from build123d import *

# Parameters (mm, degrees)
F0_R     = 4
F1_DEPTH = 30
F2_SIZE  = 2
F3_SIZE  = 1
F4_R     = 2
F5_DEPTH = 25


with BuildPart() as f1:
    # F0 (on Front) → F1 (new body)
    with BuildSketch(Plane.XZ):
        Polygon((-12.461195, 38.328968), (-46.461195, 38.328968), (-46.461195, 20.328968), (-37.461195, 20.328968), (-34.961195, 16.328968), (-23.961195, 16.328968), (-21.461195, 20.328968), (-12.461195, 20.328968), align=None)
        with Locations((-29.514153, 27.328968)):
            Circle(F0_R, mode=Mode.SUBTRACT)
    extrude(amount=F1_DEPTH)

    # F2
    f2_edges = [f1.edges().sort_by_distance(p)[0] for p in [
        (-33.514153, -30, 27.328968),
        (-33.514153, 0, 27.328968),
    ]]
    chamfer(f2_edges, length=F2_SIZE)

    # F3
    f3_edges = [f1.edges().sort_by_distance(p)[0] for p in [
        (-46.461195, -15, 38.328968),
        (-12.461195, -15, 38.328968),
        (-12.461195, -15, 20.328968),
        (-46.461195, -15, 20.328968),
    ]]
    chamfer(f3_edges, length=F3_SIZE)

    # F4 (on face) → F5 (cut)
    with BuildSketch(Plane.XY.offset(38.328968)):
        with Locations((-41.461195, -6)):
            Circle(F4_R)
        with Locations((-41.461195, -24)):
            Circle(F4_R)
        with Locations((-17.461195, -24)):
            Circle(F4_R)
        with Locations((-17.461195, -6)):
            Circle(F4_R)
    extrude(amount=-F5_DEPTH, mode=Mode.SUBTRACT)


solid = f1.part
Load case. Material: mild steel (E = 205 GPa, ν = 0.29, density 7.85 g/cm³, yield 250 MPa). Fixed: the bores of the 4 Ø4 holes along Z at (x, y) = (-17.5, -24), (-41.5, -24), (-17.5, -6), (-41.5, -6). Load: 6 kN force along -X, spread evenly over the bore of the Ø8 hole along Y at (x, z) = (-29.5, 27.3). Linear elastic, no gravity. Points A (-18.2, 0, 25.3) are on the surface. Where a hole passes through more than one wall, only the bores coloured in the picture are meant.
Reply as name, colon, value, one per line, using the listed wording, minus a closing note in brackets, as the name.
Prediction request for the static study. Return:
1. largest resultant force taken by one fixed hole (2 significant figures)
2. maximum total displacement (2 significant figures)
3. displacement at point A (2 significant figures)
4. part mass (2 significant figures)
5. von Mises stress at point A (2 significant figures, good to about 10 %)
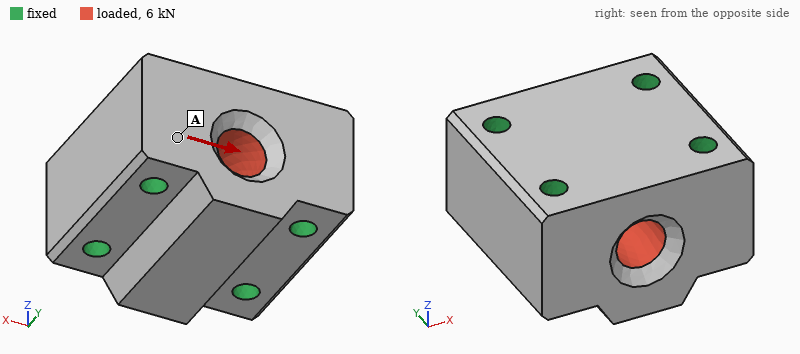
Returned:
largest resultant force taken by one fixed hole: 1.5 kN
maximum total displacement: 0.59 µm
displacement at point A: 0.12 µm
part mass: 140 g
von Mises stress at point A: 2.4 MPa
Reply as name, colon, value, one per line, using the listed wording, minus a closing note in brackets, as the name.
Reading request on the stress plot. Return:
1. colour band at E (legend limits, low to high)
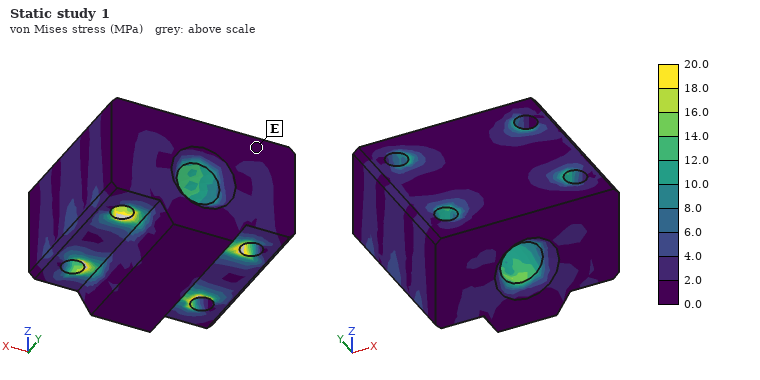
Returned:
colour band at E: 0.0 to 2.0 MPa
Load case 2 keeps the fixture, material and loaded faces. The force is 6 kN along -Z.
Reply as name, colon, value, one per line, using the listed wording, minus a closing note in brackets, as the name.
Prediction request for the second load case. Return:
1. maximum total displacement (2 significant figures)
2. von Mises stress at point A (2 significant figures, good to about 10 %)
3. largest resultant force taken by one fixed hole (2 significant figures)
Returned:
maximum total displacement: 1.1 µm
von Mises stress at point A: 4.4 MPa
largest resultant force taken by one fixed hole: 1.5 kN
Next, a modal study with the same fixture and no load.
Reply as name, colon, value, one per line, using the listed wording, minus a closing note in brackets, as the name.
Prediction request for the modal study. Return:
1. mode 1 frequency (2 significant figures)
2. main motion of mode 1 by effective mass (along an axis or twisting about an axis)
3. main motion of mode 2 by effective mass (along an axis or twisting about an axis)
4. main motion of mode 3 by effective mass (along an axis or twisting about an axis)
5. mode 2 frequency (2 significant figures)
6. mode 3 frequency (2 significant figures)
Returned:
mode 1 frequency: 53 kHz
main motion of mode 1 by effective mass: along Y
main motion of mode 2 by effective mass: along Z
main motion of mode 3 by effective mass: along Y
mode 2 frequency: 58 kHz
mode 3 frequency: 65 kHz
